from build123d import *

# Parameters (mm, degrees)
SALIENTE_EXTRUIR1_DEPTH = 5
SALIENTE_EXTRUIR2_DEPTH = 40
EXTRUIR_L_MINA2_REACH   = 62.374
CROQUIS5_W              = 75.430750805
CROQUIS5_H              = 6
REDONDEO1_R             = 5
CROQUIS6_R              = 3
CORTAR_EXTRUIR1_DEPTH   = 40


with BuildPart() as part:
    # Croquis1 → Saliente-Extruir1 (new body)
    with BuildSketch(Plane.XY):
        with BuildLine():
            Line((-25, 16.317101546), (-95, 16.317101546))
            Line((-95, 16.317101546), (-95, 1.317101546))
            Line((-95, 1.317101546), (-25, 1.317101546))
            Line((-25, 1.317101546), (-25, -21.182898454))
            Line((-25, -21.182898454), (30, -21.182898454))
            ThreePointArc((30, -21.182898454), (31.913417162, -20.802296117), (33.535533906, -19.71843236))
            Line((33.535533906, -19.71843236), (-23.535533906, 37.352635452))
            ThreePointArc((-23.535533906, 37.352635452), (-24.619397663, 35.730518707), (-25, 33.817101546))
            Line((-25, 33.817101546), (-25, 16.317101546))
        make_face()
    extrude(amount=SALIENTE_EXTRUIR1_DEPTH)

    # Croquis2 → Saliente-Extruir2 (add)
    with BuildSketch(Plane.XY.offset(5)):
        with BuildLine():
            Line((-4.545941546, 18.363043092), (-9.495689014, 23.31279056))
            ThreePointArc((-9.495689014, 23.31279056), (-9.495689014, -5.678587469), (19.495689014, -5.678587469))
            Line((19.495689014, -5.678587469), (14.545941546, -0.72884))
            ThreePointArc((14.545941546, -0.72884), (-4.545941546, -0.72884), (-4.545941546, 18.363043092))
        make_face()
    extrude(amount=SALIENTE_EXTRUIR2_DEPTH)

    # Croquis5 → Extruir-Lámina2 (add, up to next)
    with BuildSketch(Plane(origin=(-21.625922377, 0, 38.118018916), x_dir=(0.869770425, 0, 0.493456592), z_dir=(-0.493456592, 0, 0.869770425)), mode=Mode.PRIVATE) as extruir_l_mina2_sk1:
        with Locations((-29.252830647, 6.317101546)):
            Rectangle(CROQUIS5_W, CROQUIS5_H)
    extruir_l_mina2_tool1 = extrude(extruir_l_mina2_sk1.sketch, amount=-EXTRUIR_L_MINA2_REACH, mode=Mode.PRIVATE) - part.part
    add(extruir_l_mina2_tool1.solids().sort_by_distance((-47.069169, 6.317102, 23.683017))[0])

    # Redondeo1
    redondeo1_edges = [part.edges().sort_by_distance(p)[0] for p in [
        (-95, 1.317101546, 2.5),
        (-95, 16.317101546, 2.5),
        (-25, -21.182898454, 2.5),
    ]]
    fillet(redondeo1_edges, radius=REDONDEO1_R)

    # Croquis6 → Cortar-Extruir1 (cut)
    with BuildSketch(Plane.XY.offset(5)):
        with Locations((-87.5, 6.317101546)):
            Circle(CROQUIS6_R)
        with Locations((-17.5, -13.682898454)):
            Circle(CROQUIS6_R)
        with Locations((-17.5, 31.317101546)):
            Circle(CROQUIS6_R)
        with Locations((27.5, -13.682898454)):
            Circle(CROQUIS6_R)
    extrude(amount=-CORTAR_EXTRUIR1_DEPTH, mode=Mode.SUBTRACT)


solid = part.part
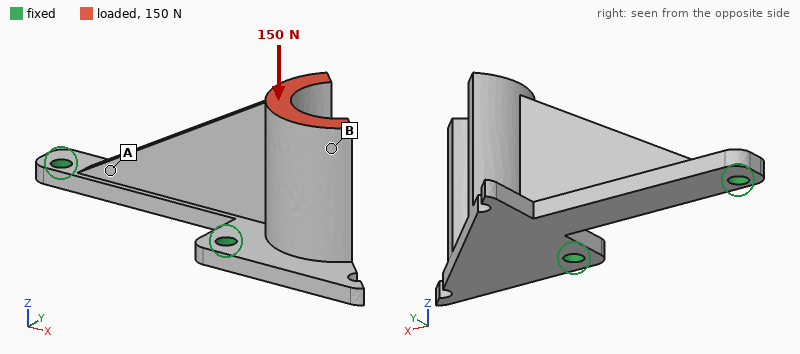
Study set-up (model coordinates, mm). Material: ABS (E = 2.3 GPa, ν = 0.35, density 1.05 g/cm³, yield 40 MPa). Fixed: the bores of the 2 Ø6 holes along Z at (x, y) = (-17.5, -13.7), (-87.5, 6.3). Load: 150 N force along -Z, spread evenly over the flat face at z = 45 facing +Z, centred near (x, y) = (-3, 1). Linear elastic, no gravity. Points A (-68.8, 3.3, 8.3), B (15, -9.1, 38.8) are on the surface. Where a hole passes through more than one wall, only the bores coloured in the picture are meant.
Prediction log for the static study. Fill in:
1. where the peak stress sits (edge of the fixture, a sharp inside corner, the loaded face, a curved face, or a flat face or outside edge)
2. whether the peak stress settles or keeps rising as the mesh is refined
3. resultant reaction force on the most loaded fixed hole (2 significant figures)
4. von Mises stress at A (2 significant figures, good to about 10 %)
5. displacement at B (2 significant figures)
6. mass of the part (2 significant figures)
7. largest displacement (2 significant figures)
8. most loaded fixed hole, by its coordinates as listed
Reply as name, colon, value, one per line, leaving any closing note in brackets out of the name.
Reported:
where the peak stress sits: edge of the fixture
whether the peak stress settles or keeps rising as the mesh is refined: keeps rising
resultant reaction force on the most loaded fixed hole: 170 N
von Mises stress at A: 4.1 MPa
displacement at B: 0.92 mm
mass of the part: 38 g
largest displacement: 1.2 mm
most loaded fixed hole, by its coordinates as listed: (-17.5, -13.7)
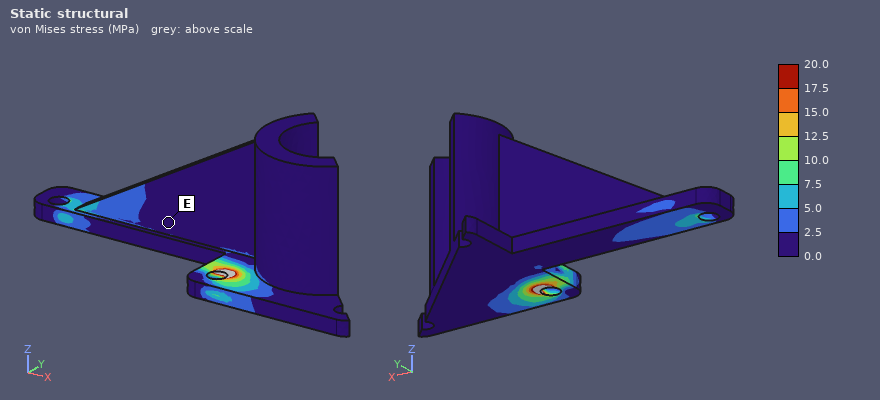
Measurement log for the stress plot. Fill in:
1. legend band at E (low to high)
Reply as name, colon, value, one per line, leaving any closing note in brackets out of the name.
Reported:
legend band at E: 0.0 to 2.5 MPa
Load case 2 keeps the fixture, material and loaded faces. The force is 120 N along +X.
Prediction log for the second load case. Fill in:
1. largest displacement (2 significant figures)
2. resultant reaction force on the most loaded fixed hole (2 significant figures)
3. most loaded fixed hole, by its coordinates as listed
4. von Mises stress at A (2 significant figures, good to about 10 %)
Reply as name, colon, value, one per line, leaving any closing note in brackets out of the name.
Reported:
largest displacement: 0.89 mm
resultant reaction force on the most loaded fixed hole: 130 N
most loaded fixed hole, by its coordinates as listed: (-87.5, 6.3)
von Mises stress at A: 5.3 MPa
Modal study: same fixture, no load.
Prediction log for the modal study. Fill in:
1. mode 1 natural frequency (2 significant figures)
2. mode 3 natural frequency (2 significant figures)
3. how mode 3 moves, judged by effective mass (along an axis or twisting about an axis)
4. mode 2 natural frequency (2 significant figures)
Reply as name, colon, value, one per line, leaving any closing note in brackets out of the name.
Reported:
mode 1 natural frequency: 320 Hz
mode 3 natural frequency: 1400 Hz
how mode 3 moves, judged by effective mass: along Z
mode 2 natural frequency: 1000 Hz
